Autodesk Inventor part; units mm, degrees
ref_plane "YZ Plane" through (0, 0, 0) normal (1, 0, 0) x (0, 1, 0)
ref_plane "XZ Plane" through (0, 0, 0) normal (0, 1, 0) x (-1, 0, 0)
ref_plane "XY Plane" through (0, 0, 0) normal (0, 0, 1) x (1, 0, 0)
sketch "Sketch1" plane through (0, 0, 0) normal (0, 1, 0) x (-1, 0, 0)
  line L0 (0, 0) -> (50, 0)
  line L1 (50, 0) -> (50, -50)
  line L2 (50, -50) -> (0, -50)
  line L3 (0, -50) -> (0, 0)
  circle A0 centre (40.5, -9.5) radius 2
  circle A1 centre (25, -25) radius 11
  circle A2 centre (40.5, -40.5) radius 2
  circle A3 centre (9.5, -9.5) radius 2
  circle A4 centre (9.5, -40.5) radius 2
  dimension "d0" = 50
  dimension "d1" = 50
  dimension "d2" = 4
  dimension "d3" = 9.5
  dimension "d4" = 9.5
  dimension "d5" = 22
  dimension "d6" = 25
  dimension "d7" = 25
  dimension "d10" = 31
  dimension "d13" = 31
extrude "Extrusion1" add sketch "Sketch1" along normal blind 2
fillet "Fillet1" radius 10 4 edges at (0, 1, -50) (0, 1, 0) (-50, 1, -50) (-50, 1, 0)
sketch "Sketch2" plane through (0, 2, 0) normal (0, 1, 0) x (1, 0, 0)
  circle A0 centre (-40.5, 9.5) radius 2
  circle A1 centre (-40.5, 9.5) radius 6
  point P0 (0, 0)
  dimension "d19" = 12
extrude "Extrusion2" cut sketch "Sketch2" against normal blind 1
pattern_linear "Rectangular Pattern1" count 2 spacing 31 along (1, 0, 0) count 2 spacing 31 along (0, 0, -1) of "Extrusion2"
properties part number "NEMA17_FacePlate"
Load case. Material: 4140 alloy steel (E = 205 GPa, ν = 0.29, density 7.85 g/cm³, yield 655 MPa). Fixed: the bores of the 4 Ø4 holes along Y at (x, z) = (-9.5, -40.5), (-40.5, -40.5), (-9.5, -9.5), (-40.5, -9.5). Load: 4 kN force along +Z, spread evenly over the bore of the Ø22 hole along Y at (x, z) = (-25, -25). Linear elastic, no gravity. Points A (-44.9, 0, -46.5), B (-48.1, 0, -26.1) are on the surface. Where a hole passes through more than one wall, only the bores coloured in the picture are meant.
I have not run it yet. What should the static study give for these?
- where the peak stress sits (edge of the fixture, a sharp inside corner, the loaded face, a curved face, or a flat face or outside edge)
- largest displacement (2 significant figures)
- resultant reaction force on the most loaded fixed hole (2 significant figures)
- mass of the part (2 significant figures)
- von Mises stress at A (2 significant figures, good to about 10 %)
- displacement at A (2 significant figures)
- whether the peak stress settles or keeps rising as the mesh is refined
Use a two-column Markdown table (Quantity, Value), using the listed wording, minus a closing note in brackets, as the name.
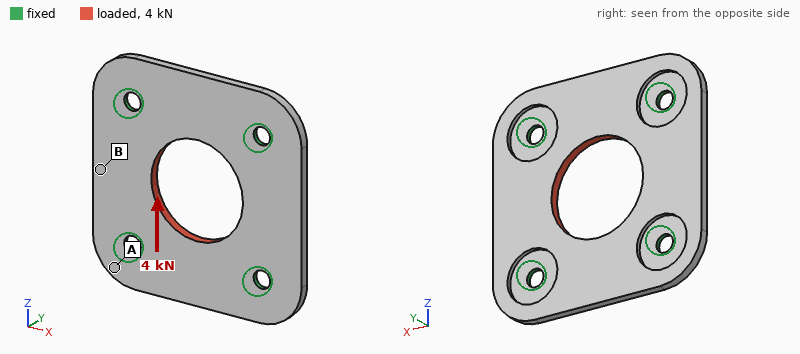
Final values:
| Quantity | Value |
|---|---|
| where the peak stress sits | edge of the fixture |
| largest displacement | 10 µm |
| resultant reaction force on the most loaded fixed hole | 1.0 kN |
| mass of the part | 28 g |
| von Mises stress at A | 30 MPa |
| displacement at A | 3.1 µm |
| whether the peak stress settles or keeps rising as the mesh is refined | keeps rising |
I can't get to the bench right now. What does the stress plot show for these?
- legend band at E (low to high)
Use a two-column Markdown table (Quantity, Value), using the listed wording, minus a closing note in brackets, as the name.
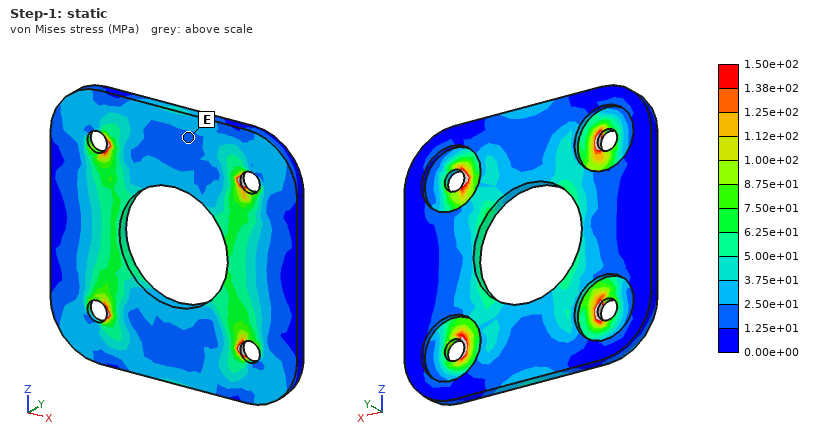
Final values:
| Quantity | Value |
|---|---|
| legend band at E | 1.25e+01 to 2.50e+01 MPa |
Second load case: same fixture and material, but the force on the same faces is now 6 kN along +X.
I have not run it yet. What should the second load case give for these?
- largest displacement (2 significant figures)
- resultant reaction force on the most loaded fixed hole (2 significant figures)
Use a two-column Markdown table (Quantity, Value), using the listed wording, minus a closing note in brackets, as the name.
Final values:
| Quantity | Value |
|---|---|
| largest displacement | 16 µm |
| resultant reaction force on the most loaded fixed hole | 1.5 kN |
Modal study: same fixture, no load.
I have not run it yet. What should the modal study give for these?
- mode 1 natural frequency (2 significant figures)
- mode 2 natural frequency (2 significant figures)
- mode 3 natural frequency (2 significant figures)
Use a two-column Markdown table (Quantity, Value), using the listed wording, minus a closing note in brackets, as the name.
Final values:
| Quantity | Value |
|---|---|
| mode 1 natural frequency | 6600 Hz |
| mode 2 natural frequency | 7500 Hz |
| mode 3 natural frequency | 7500 Hz |
